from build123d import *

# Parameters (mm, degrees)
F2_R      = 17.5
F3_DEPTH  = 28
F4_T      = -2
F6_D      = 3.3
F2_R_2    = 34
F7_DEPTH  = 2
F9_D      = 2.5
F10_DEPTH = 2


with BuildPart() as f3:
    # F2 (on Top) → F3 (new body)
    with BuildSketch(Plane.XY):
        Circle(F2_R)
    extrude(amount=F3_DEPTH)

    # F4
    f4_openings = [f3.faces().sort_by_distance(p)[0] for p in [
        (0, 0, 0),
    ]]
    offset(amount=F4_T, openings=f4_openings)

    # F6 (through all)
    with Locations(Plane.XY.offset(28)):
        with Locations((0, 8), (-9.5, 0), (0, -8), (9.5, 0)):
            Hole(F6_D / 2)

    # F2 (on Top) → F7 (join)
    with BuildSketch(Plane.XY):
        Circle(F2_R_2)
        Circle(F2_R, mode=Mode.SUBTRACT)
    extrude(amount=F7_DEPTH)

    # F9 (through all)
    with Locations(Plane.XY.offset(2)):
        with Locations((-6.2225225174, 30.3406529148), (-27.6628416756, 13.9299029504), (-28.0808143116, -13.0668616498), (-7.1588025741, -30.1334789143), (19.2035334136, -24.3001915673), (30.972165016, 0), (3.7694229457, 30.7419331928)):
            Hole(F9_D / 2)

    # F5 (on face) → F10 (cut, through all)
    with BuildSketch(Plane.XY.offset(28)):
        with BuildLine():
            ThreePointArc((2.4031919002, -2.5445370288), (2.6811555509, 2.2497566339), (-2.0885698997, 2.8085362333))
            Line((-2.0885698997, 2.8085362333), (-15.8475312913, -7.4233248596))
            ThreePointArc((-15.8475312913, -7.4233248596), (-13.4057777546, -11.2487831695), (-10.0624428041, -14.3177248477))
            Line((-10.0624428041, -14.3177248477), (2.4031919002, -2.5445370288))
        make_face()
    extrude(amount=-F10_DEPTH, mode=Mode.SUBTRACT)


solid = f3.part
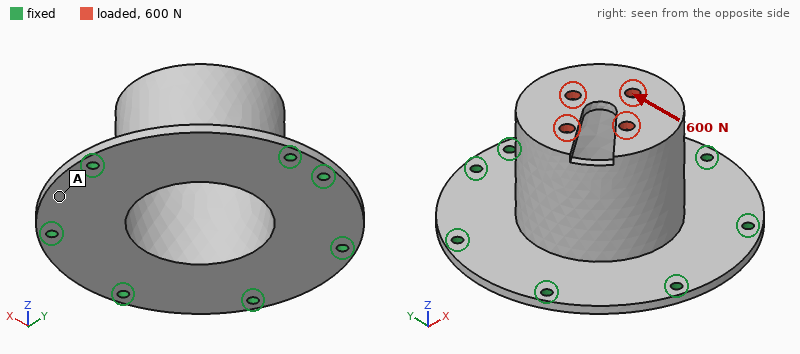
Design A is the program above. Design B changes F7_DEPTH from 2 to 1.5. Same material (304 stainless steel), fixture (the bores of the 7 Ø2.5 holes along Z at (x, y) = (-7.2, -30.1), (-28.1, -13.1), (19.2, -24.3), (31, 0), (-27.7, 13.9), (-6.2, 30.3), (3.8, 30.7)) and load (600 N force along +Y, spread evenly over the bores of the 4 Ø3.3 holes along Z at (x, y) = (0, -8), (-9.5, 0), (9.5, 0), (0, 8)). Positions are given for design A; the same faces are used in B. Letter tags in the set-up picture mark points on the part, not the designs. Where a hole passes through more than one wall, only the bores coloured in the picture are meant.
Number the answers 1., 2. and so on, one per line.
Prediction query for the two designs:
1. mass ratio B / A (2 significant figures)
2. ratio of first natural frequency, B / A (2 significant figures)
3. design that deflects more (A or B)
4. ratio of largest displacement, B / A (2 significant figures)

1. 0.89
2. 0.73
3. B
4. 1.9
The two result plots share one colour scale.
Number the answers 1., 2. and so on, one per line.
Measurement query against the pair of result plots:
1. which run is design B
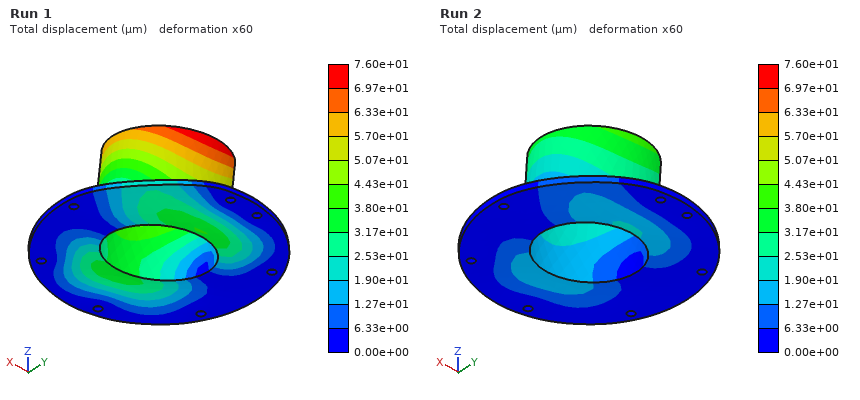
1. Run 1
